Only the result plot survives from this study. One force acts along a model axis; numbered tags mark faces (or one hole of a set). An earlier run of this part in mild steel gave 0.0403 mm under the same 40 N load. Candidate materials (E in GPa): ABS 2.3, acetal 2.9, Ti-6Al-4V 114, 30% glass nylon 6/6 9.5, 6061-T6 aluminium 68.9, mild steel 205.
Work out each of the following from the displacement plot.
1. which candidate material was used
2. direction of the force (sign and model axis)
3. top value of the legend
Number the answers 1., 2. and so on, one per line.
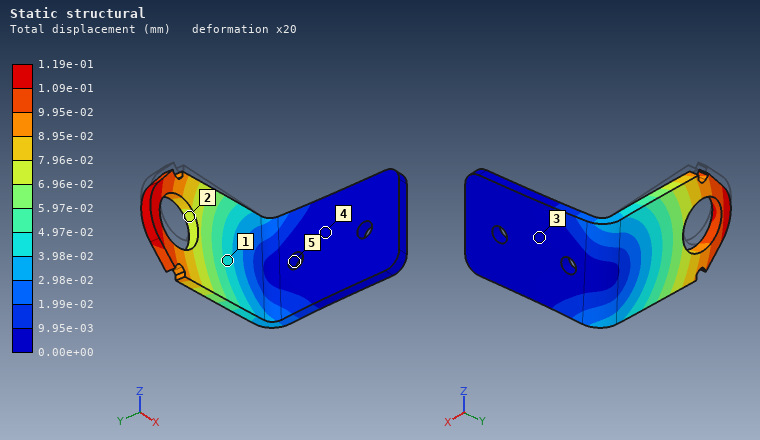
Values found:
1. 6061-T6 aluminium
2. -Z
3. 1.19e-01 mm
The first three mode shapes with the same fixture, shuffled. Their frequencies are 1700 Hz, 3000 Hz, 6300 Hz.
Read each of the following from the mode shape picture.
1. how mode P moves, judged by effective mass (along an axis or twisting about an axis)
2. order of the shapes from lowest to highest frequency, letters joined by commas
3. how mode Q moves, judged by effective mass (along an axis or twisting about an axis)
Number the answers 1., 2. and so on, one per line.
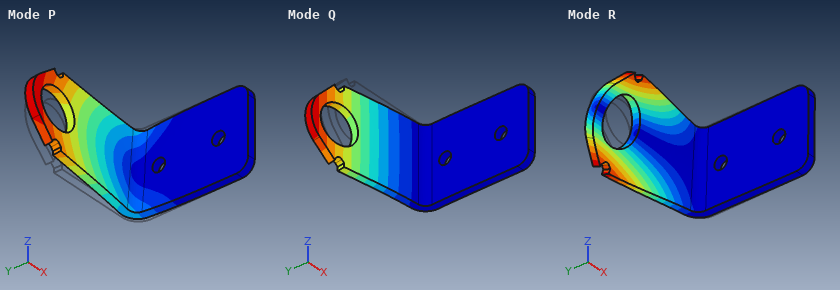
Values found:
1. along Z
2. Q, P, R
3. along Y
